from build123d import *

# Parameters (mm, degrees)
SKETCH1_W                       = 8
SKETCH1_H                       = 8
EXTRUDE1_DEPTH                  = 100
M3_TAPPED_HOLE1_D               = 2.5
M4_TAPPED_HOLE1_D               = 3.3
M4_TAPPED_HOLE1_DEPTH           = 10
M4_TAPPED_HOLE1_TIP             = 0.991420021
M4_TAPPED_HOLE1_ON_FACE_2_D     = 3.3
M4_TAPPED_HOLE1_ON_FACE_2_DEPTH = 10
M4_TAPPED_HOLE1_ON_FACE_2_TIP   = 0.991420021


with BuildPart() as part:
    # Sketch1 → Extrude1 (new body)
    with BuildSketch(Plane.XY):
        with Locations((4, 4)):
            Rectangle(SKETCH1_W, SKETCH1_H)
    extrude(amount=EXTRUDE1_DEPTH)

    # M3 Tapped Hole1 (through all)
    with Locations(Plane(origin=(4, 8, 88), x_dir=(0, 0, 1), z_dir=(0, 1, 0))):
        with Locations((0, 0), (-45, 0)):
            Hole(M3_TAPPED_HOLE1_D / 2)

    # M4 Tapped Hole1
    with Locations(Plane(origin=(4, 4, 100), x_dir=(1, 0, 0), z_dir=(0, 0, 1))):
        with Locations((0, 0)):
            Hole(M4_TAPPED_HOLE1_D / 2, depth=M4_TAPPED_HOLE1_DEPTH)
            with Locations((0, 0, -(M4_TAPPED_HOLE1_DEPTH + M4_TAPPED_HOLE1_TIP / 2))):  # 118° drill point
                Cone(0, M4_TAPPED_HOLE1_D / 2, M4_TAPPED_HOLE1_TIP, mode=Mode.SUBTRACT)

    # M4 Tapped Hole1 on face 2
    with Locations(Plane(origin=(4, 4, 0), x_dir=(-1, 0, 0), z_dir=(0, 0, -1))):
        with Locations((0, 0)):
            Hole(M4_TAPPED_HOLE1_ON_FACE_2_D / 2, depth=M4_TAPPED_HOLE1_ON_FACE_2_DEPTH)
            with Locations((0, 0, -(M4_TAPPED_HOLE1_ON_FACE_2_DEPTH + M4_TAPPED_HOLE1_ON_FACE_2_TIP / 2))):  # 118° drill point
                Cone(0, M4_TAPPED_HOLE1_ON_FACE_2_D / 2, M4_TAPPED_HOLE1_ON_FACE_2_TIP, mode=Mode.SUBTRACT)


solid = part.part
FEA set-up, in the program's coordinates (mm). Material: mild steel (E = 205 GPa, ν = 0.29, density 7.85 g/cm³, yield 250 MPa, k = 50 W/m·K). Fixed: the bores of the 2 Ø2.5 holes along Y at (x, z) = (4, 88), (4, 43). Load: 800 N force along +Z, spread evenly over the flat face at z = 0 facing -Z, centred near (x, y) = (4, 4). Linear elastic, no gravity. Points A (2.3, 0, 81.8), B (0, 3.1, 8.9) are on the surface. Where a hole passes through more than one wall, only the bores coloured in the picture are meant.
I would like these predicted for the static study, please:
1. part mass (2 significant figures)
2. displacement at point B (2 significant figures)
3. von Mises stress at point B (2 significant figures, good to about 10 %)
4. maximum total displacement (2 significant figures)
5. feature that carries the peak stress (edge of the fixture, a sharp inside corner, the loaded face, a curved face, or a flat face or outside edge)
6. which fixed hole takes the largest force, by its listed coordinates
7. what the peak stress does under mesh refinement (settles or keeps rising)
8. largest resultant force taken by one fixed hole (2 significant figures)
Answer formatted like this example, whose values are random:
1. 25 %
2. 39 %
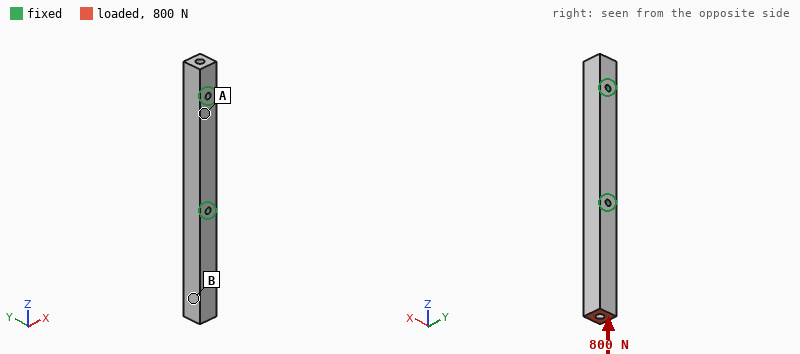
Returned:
1. 48 g
2. 2.1 µm
3. 14 MPa
4. 2.8 µm
5. edge of the fixture
6. (4, 43)
7. keeps rising
8. 780 N
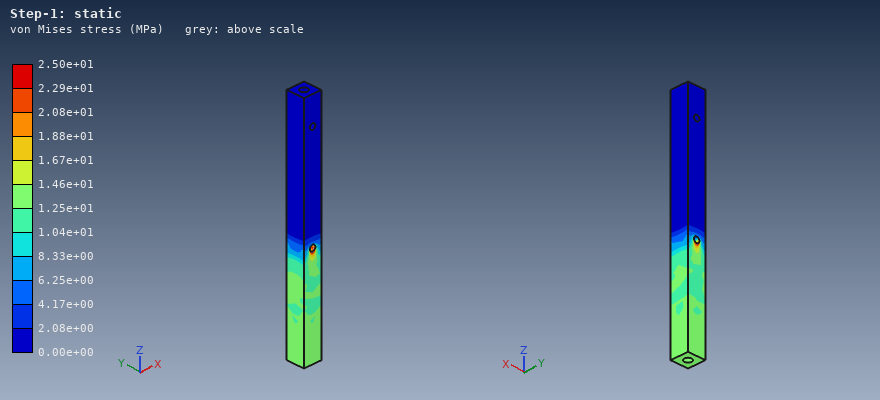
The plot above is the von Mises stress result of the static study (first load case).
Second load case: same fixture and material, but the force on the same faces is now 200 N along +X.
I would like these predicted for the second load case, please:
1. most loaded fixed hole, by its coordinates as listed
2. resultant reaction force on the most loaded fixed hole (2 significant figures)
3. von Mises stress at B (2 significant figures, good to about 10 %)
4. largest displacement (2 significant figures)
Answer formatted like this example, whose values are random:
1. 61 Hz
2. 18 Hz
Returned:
1. (4, 43)
2. 270 N
3. 21 MPa
4. 95 µm
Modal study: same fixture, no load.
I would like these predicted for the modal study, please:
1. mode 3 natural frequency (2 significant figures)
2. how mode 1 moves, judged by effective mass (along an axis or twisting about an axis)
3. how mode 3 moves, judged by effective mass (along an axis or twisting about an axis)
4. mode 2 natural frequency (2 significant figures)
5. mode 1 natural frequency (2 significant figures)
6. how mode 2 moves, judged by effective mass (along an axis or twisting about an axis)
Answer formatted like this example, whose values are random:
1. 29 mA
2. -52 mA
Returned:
1. 15 kHz
2. along X
3. along X
4. 3600 Hz
5. 3200 Hz
6. along Y
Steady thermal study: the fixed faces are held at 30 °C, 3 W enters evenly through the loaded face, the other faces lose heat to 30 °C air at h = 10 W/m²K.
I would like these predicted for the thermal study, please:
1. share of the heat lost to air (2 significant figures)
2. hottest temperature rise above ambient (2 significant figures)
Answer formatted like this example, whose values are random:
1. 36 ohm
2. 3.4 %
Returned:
1. 9.8 %
2. 39 K
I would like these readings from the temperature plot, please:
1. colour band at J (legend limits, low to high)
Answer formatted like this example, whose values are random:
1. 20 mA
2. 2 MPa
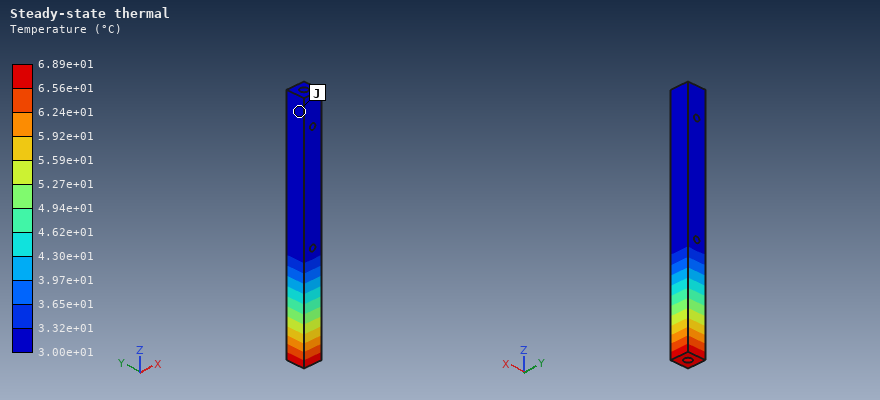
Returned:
1. 3.00e+01 to 3.32e+01 °C
